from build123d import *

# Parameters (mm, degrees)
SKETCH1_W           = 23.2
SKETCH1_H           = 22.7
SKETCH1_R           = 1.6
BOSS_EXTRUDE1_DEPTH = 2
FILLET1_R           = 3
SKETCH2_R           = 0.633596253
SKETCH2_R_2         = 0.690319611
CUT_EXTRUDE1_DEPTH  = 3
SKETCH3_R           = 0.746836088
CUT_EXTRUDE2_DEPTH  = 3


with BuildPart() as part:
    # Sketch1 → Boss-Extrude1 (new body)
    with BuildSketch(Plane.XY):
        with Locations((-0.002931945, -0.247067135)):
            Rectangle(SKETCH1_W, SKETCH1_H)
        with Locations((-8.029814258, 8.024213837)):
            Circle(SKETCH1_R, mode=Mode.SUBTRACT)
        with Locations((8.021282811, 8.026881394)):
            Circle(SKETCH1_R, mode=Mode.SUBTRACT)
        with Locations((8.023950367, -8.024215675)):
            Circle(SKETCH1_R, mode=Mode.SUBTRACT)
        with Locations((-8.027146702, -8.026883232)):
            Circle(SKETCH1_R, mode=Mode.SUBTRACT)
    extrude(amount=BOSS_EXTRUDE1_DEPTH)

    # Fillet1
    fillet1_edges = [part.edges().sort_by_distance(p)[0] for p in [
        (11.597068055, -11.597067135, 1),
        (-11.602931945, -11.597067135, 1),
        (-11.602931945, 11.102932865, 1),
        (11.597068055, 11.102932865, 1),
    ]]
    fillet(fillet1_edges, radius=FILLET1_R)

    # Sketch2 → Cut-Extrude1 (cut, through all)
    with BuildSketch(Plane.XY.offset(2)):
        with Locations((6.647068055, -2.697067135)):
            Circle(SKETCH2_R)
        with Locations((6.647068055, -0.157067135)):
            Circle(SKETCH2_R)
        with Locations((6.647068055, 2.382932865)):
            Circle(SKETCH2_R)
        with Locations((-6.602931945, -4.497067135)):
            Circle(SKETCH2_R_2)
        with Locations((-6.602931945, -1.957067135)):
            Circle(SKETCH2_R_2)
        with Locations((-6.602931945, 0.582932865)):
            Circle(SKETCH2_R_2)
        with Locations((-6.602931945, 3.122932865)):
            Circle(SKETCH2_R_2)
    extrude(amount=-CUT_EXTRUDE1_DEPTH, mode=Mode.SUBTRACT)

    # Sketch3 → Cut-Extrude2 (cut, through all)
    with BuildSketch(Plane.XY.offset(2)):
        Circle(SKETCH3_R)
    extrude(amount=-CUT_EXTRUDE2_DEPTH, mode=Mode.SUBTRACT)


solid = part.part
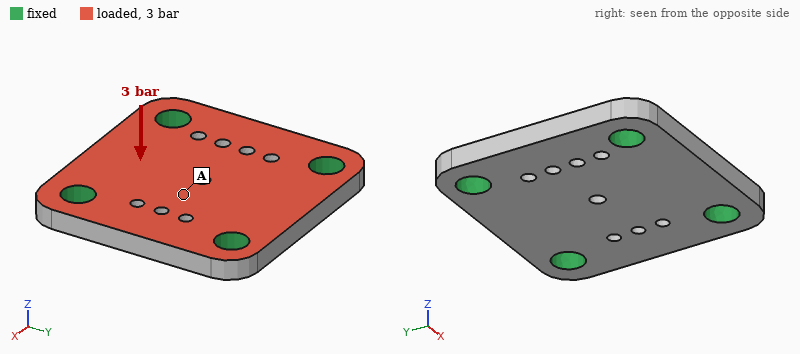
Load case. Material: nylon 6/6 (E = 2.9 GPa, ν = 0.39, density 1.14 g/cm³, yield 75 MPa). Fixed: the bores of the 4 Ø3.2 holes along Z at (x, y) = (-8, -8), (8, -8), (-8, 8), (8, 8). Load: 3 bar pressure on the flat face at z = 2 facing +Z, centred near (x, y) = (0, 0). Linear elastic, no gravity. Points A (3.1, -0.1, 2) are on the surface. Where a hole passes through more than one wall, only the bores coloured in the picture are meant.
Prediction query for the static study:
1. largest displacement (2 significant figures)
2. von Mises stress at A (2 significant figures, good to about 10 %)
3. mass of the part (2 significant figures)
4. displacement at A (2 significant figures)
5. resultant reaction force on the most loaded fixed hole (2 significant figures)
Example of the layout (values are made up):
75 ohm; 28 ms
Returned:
44 µm; 4.1 MPa; 1.1 g; 38 µm; 37 N
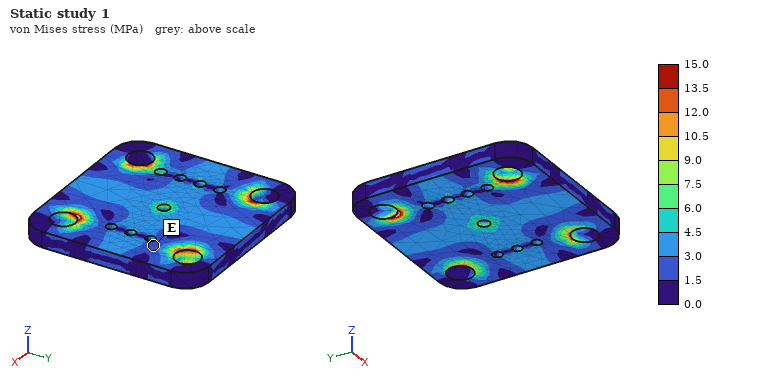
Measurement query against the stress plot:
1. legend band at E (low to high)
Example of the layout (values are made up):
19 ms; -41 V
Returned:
1.5 to 3.0 MPa
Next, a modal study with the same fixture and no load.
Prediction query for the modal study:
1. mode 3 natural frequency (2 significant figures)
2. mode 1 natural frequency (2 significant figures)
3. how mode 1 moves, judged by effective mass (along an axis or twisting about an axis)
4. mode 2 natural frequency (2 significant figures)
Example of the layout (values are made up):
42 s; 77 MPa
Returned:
16 kHz; 11 kHz; along Z; 16 kHz
